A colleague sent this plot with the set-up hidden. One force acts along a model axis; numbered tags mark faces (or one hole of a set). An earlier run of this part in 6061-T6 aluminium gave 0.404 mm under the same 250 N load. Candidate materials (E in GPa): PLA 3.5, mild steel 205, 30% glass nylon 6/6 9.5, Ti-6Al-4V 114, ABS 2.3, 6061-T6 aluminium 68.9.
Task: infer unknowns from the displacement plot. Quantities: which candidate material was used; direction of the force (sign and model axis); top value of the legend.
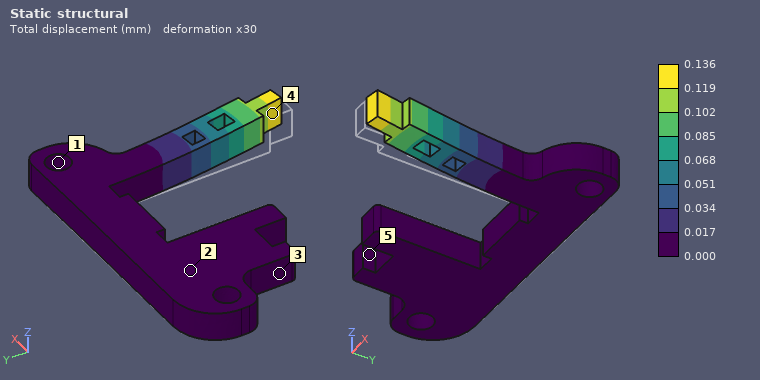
mild steel
+X
0.136 mm
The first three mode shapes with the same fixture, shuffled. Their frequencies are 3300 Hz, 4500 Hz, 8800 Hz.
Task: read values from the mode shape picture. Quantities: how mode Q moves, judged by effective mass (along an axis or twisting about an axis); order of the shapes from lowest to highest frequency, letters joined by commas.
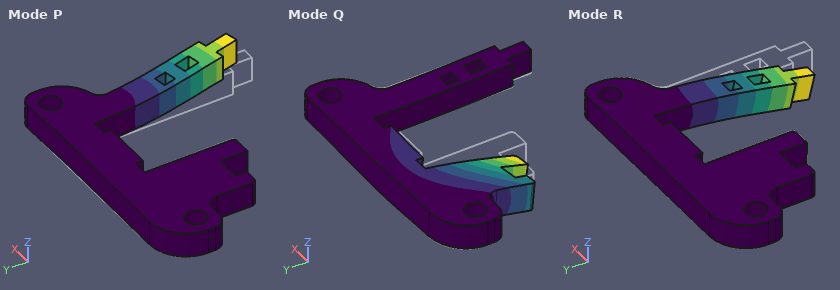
along Z
R, P, Q
